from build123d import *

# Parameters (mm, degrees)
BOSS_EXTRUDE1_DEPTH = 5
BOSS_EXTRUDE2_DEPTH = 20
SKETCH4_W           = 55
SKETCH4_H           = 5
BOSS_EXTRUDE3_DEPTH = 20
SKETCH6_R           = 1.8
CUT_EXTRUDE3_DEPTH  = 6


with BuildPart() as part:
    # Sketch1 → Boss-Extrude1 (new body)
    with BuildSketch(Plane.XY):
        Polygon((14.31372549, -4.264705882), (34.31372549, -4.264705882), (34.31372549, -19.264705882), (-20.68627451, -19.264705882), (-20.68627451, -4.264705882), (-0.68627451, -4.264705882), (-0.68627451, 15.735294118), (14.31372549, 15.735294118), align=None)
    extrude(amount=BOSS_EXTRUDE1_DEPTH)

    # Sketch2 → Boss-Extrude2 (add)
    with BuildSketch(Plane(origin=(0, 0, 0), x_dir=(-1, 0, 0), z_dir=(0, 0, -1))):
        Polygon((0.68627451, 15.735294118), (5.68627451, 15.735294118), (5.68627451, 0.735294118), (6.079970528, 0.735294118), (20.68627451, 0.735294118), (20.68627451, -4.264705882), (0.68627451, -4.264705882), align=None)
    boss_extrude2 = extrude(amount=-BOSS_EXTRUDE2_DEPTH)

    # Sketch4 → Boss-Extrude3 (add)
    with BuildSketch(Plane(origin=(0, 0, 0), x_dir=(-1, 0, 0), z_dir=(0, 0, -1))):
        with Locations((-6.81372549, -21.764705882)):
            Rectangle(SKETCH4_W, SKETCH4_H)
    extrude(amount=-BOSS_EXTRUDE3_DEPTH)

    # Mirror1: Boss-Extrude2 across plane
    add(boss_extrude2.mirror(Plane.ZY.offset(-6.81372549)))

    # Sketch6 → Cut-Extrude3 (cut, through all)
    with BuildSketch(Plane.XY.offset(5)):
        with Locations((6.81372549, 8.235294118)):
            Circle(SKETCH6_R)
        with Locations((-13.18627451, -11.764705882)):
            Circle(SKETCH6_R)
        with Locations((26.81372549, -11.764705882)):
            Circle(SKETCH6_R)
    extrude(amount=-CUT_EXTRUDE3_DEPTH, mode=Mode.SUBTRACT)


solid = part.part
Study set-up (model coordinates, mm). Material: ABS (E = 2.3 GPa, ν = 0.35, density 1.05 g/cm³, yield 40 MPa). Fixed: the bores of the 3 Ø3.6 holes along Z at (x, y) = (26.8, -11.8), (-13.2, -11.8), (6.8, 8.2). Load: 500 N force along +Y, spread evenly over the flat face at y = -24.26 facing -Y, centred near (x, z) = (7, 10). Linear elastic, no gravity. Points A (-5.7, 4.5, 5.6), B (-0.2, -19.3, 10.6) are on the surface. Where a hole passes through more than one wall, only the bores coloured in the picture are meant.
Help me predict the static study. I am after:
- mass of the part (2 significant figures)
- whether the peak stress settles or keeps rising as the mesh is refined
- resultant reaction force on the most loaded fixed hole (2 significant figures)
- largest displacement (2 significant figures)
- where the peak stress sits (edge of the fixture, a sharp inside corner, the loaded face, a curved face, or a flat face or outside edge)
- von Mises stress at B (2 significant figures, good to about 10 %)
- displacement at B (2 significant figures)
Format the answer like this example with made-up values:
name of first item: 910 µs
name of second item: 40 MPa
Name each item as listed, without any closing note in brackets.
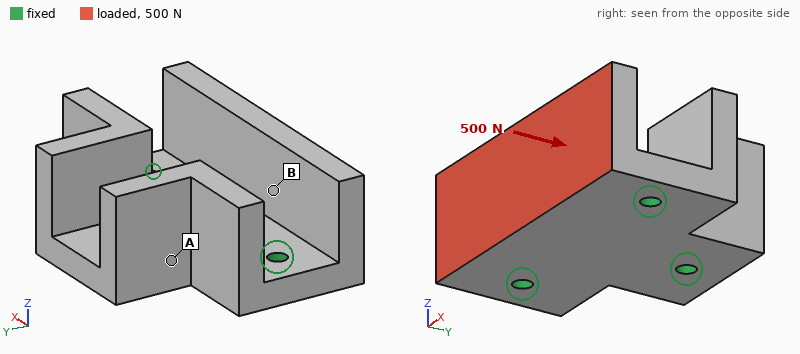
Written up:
mass of the part: 19 g
whether the peak stress settles or keeps rising as the mesh is refined: keeps rising
resultant reaction force on the most loaded fixed hole: 180 N
largest displacement: 0.74 mm
where the peak stress sits: edge of the fixture
von Mises stress at B: 4.7 MPa
displacement at B: 0.31 mm
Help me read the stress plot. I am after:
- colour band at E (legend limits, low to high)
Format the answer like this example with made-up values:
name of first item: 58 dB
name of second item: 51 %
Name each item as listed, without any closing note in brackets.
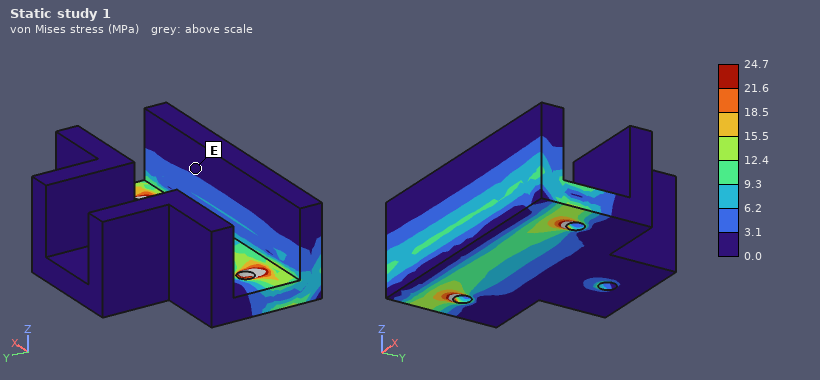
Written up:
colour band at E: 0.0 to 3.1 MPa
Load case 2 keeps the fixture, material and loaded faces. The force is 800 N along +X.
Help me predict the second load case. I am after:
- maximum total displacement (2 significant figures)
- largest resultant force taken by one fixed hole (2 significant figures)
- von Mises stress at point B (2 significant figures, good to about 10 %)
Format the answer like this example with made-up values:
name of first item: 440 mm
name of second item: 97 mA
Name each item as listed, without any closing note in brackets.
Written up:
maximum total displacement: 0.18 mm
largest resultant force taken by one fixed hole: 480 N
von Mises stress at point B: 4.2 MPa
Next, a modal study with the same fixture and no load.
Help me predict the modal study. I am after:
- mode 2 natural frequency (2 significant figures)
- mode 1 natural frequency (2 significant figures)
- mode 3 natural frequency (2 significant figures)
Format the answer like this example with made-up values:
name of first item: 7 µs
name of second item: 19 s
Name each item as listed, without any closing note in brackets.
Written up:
mode 2 natural frequency: 2800 Hz
mode 1 natural frequency: 1900 Hz
mode 3 natural frequency: 2800 Hz
